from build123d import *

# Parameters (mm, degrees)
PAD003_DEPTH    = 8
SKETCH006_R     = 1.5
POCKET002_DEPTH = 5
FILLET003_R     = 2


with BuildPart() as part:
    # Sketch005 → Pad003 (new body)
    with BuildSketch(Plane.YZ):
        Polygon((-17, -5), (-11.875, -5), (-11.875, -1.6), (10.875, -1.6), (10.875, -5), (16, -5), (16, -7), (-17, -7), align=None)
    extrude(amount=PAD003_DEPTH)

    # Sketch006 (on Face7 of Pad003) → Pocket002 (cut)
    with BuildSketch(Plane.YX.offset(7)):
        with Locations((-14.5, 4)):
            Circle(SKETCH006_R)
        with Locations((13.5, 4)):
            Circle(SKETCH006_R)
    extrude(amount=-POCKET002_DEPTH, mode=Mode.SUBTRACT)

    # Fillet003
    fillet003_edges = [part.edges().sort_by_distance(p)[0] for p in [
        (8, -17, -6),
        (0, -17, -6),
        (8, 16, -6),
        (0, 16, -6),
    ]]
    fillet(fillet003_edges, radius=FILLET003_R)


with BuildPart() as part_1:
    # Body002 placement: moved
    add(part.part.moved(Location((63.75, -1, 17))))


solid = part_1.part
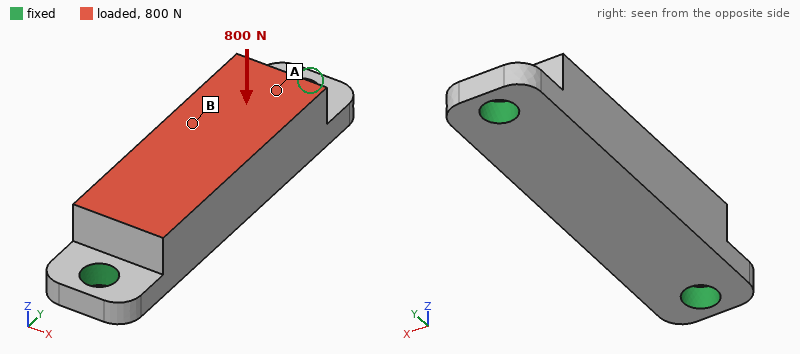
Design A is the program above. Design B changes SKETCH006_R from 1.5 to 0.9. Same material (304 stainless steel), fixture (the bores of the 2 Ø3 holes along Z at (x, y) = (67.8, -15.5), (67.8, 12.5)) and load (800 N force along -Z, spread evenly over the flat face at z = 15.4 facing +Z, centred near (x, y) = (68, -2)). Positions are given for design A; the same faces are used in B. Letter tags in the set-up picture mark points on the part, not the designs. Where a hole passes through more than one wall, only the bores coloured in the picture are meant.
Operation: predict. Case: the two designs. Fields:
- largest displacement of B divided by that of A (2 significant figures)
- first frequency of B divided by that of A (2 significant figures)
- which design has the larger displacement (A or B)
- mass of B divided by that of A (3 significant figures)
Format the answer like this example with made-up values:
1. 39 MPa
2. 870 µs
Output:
1. 1.3
2. 0.80
3. B
4. 1.02
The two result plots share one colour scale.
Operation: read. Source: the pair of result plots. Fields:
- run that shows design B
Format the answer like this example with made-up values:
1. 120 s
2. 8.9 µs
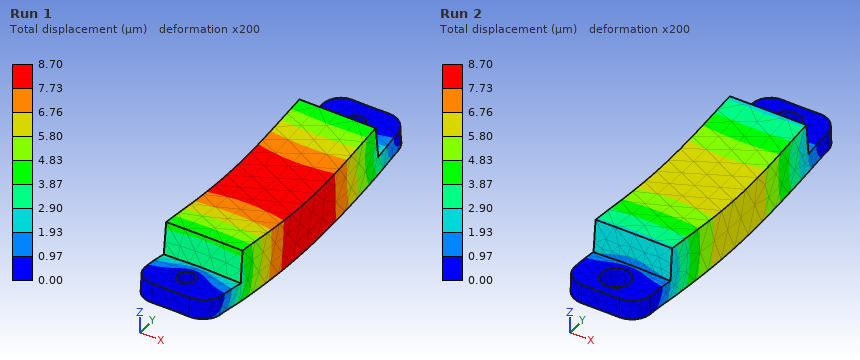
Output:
1. Run 1
